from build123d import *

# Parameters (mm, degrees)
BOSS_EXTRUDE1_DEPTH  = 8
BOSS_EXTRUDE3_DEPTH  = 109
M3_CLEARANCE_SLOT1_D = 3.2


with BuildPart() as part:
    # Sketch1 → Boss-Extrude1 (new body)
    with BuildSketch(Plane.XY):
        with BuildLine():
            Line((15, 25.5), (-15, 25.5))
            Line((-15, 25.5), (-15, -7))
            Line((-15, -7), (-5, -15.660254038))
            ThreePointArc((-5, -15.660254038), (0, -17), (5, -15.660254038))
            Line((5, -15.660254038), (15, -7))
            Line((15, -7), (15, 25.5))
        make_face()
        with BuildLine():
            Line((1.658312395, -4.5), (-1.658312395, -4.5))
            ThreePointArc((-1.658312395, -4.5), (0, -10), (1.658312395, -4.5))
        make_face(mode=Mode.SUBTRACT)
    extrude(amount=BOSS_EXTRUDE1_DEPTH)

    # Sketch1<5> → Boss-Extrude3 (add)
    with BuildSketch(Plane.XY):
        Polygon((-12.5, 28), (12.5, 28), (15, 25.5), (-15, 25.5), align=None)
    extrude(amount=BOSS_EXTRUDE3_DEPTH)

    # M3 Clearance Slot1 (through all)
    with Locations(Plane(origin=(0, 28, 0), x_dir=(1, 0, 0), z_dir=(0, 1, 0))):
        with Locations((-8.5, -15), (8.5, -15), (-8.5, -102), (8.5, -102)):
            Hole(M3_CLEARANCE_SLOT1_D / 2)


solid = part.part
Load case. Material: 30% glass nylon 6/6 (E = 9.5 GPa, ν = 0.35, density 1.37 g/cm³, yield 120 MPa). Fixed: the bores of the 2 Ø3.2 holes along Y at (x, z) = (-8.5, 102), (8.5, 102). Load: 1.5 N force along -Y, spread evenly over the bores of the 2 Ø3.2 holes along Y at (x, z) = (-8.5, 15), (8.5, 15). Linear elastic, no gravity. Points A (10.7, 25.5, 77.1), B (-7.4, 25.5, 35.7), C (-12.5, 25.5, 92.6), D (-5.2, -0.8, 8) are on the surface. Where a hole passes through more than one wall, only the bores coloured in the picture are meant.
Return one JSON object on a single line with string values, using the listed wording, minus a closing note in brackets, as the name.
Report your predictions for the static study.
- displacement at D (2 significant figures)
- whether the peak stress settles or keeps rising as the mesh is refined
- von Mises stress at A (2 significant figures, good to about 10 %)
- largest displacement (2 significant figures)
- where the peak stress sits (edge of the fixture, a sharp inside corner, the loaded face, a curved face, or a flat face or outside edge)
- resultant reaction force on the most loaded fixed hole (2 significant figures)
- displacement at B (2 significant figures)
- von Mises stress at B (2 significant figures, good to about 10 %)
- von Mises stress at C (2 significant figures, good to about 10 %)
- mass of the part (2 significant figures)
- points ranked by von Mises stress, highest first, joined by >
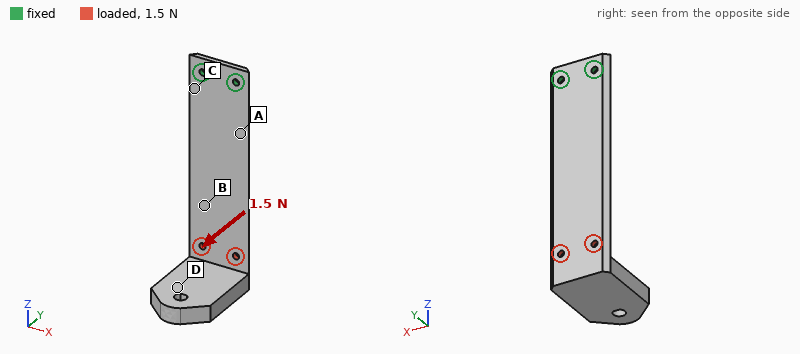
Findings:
{"displacement at D": "1.2 mm", "whether the peak stress settles or keeps rising as the mesh is refined": "keeps rising", "von Mises stress at A": "3.2 MPa", "largest displacement": "1.4 mm", "where the peak stress sits": "edge of the fixture", "resultant reaction force on the most loaded fixed hole": "1.1 N", "displacement at B": "0.61 mm", "von Mises stress at B": "1.1 MPa", "von Mises stress at C": "4.0 MPa", "mass of the part": "23 g", "points ranked by von Mises stress, highest first, joined by >": "C > A > B > D"}
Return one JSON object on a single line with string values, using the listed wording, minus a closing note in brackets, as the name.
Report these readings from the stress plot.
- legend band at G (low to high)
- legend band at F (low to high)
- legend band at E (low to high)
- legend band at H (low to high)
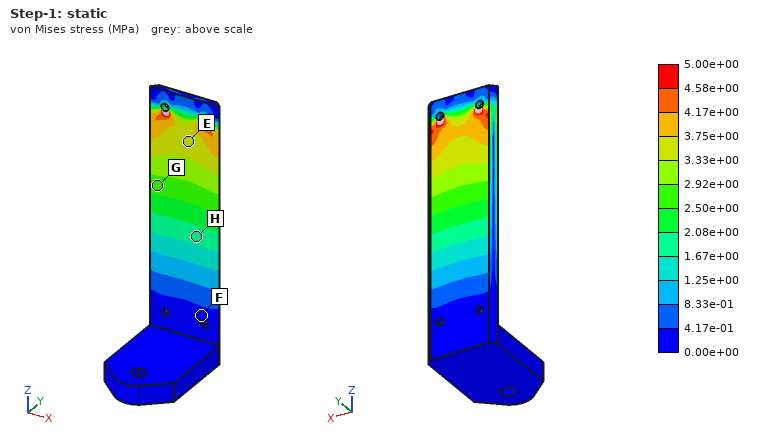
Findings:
{"legend band at G": "2.50e+00 to 2.92e+00 MPa", "legend band at F": "0.00e+00 to 4.17e-01 MPa", "legend band at E": "3.33e+00 to 3.75e+00 MPa", "legend band at H": "1.67e+00 to 2.08e+00 MPa"}
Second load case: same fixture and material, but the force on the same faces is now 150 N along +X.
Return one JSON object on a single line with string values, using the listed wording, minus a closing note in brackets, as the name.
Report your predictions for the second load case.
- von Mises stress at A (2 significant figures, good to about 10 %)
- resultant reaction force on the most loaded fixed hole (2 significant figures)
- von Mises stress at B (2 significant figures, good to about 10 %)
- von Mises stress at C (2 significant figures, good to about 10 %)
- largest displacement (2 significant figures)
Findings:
{"von Mises stress at A": "23 MPa", "resultant reaction force on the most loaded fixed hole": "710 N", "von Mises stress at B": "6.9 MPa", "von Mises stress at C": "31 MPa", "largest displacement": "1.2 mm"}
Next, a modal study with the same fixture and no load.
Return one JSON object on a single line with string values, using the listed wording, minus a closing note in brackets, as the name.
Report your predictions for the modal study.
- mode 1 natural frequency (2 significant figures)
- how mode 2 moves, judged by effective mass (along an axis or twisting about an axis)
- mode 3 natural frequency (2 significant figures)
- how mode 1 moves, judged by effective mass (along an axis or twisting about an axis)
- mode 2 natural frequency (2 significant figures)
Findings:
{"mode 1 natural frequency": "41 Hz", "how mode 2 moves, judged by effective mass": "along X", "mode 3 natural frequency": "230 Hz", "how mode 1 moves, judged by effective mass": "along Y", "mode 2 natural frequency": "130 Hz"}
